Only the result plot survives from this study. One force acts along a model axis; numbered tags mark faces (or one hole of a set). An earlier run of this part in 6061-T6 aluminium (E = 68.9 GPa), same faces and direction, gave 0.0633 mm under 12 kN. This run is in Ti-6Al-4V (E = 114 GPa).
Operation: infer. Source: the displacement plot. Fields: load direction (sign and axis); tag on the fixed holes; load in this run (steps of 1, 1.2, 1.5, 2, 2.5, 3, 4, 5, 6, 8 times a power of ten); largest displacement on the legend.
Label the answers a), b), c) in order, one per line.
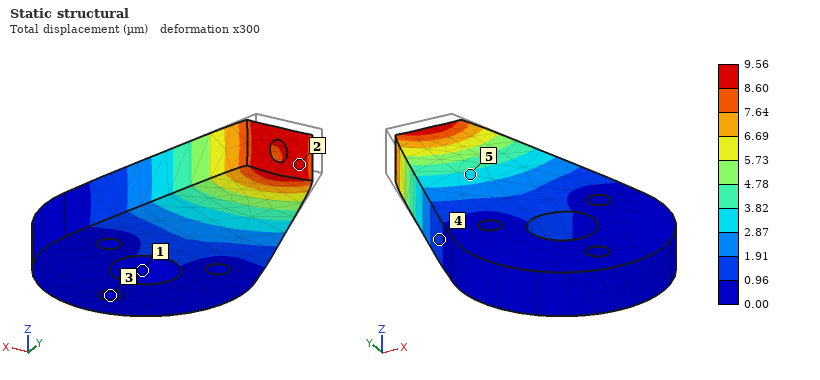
a) -Y
b) 3
c) 3 kN
d) 9.56 µm
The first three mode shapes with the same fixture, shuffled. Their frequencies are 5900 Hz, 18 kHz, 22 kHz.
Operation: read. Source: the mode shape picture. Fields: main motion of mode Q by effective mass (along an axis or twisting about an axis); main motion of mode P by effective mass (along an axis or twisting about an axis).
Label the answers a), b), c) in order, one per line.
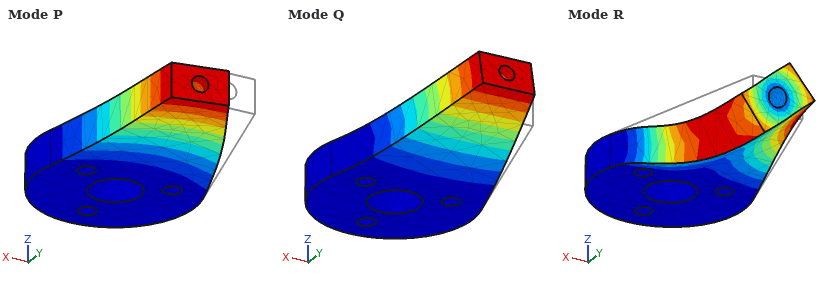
a) along Z
b) along X
